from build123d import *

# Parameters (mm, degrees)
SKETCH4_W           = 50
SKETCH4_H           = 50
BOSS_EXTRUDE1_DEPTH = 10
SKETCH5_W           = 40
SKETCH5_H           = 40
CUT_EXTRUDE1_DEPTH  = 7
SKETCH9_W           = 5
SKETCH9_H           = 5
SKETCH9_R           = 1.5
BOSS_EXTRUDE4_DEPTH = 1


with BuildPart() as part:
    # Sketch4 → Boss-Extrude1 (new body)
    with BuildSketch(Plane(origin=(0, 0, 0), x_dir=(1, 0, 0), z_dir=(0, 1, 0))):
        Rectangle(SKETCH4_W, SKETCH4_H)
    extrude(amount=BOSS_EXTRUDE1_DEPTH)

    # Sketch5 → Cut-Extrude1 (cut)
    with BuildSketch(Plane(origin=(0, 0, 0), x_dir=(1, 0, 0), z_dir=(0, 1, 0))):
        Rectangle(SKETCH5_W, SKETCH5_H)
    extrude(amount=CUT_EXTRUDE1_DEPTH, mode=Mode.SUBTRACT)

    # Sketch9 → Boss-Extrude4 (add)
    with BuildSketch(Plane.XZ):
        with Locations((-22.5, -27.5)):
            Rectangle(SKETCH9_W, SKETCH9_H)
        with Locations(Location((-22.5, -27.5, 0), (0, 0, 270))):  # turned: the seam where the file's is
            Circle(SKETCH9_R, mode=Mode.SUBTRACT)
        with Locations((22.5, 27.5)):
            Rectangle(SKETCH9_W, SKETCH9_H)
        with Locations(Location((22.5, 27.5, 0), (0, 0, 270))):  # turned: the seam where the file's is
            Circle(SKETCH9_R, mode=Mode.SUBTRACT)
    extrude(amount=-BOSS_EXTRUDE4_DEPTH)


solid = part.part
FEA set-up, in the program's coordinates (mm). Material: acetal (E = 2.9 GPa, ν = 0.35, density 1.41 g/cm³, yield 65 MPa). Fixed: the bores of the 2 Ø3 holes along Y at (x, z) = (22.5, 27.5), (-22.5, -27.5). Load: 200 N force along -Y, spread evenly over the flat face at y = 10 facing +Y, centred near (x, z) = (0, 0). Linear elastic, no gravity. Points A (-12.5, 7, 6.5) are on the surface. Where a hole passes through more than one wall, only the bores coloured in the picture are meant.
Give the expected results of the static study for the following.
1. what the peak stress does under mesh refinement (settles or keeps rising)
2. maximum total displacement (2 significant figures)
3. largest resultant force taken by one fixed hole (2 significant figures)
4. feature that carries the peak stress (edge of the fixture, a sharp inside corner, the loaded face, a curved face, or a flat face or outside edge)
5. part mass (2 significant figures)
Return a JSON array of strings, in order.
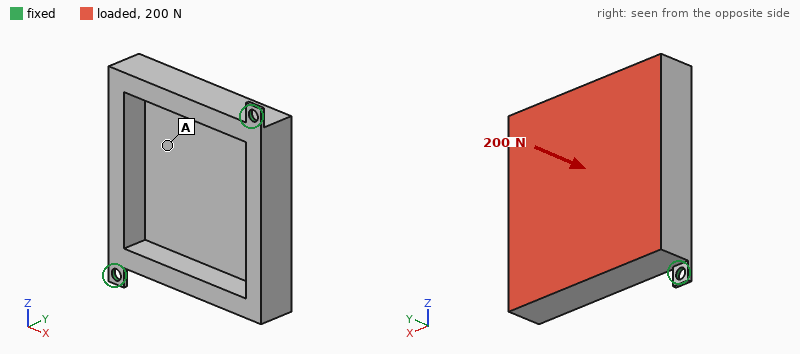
["keeps rising", "0.50 mm", "200 N", "edge of the fixture", "20 g"]
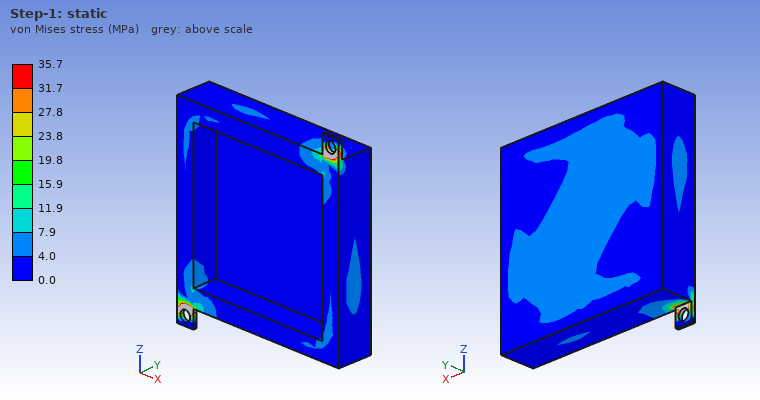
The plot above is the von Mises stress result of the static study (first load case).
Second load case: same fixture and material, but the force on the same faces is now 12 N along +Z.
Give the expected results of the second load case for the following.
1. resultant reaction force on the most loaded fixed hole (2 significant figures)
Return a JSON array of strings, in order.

["6.3 N"]
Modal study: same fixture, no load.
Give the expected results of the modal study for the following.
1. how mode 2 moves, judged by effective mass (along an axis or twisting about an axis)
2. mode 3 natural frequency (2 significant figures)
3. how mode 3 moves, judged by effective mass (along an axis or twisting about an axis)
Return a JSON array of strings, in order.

["along Y", "1700 Hz", "along X"]
